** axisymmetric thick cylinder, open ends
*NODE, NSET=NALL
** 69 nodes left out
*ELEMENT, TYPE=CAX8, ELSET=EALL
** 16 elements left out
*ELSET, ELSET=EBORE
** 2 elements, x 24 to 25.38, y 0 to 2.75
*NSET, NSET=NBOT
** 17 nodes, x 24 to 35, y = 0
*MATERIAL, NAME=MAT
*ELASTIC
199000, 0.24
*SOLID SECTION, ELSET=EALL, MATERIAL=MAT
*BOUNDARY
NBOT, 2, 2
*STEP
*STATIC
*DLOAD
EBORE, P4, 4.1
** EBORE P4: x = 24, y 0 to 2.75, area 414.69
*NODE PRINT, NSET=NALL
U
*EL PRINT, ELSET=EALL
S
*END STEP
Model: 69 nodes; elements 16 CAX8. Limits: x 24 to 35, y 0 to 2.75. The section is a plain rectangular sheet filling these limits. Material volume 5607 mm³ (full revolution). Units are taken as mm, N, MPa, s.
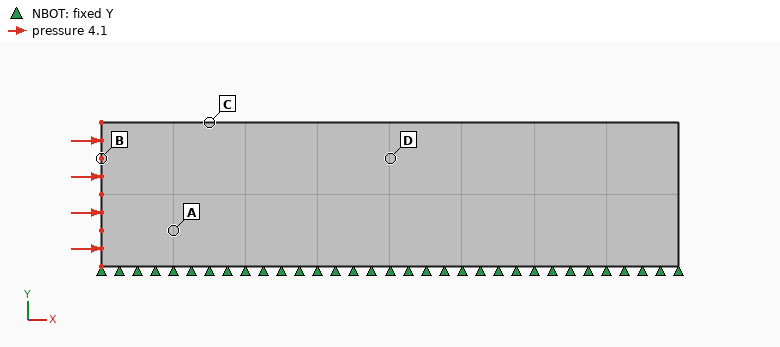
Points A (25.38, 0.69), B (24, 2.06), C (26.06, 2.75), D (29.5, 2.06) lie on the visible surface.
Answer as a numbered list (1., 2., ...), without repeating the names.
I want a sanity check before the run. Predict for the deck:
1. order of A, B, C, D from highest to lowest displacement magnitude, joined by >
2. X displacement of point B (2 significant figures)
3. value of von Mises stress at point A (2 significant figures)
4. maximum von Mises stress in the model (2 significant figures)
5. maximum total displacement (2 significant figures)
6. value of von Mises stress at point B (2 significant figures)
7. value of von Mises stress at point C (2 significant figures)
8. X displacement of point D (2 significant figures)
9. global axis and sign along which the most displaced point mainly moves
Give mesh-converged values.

1. B > A > C > D
2. 0.0015 mm
3. 13 MPa
4. 14 MPa
5. 0.0015 mm
6. 14 MPa
7. 12 MPa
8. 0.0014 mm
9. +X
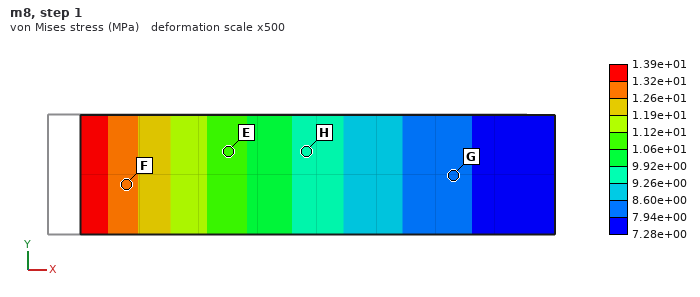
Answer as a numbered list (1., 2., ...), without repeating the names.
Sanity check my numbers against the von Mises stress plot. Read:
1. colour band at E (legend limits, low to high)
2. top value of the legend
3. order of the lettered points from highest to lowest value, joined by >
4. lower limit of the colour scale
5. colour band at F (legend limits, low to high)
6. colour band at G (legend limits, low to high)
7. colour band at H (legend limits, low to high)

1. 1.06e+01 to 1.12e+01 MPa
2. 1.39e+01 MPa
3. F > E > H > G
4. 7.28e+00 MPa
5. 1.26e+01 to 1.32e+01 MPa
6. 7.94e+00 to 8.60e+00 MPa
7. 9.26e+00 to 9.92e+00 MPa
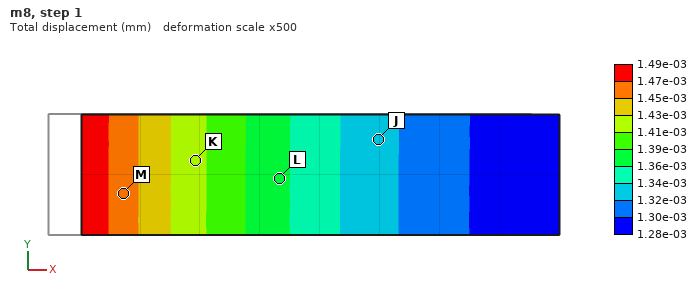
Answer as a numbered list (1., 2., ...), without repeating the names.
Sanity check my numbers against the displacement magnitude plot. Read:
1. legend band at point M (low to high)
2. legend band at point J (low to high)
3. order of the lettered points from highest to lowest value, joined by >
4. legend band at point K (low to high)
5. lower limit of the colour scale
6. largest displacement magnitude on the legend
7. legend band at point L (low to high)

1. 1.45e-03 to 1.47e-03 mm
2. 1.32e-03 to 1.34e-03 mm
3. M > K > L > J
4. 1.41e-03 to 1.43e-03 mm
5. 1.28e-03 mm
6. 1.49e-03 mm
7. 1.36e-03 to 1.39e-03 mm
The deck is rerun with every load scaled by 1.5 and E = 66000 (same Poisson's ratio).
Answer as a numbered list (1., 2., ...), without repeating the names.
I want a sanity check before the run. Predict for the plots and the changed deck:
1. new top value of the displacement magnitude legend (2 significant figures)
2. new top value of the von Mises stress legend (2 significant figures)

1. 0.0067 mm
2. 21 MPa
